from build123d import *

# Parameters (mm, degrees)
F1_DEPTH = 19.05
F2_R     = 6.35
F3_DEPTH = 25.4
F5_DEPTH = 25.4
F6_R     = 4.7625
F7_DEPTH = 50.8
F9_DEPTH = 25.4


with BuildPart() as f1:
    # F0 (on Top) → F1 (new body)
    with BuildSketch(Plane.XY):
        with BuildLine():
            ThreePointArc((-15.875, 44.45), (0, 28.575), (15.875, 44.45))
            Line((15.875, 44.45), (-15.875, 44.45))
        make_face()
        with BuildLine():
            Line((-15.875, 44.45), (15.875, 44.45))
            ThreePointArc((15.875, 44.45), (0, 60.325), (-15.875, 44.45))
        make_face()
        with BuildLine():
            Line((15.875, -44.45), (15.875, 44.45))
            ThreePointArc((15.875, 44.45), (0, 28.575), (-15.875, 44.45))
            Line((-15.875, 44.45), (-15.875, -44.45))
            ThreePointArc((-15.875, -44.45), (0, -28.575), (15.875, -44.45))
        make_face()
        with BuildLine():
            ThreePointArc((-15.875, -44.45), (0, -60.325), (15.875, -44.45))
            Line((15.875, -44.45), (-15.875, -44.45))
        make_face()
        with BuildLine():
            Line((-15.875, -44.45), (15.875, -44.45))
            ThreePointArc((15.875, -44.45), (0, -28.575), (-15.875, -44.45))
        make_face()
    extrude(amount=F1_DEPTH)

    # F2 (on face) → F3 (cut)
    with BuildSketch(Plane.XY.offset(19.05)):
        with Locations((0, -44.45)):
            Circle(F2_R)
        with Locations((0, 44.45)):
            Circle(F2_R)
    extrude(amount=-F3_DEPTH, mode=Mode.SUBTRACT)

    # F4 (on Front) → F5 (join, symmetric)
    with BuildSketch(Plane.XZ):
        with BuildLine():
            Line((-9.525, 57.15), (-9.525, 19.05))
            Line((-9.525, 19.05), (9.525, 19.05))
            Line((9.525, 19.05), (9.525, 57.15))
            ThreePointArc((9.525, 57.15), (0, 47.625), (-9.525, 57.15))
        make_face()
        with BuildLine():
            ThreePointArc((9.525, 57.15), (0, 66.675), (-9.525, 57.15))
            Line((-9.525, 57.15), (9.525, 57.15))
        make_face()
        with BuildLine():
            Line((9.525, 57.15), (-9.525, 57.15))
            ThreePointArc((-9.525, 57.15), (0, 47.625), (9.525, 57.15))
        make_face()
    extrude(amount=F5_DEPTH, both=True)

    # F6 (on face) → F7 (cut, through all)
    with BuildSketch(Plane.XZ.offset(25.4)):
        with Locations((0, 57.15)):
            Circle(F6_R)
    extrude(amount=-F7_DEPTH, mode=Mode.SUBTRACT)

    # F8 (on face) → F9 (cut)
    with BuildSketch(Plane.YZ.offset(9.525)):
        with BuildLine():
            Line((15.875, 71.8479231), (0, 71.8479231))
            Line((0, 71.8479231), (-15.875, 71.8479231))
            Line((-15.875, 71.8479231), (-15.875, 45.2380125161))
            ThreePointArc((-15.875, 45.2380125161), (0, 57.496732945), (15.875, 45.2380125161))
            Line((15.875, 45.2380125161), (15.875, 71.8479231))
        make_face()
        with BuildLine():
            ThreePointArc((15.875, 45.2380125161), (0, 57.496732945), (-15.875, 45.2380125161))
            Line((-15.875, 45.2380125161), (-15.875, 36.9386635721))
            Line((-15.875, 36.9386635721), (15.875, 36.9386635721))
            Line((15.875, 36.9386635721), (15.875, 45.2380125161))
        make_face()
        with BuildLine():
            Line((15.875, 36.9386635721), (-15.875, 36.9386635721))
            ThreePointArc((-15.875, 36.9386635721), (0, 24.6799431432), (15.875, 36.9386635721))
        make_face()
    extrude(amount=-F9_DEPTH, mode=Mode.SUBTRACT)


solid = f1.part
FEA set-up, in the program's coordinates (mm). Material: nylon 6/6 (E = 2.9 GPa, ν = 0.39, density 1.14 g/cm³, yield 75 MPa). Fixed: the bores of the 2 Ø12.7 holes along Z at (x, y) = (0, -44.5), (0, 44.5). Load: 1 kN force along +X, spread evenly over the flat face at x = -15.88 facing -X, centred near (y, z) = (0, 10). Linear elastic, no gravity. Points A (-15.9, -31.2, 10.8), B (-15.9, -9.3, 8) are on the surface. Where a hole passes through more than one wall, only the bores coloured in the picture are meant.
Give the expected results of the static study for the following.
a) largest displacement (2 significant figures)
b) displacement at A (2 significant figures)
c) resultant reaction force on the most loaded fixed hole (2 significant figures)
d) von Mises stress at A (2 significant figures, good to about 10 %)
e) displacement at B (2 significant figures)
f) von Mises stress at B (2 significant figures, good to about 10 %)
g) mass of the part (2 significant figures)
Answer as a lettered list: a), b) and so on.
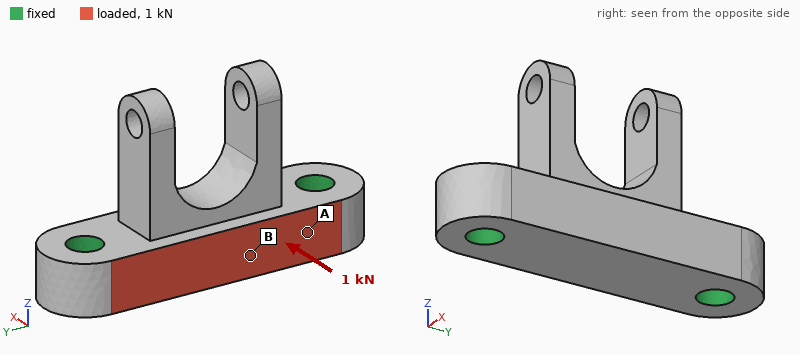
a) 36 µm
b) 17 µm
c) 500 N
d) 0.62 MPa
e) 32 µm
f) 1.4 MPa
g) 96 g
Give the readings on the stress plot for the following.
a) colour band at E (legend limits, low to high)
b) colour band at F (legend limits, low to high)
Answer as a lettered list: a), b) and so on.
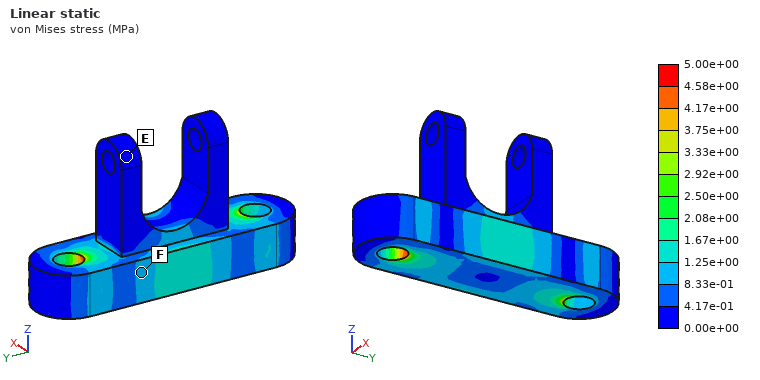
a) 0.00e+00 to 4.17e-01 MPa
b) 8.33e-01 to 1.25e+00 MPa
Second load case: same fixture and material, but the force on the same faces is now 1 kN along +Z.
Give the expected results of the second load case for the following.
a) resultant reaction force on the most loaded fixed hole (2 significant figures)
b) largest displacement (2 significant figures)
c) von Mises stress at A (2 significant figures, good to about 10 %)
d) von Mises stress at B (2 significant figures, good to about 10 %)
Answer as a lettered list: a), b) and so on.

a) 500 N
b) 0.14 mm
c) 4.1 MPa
d) 1.5 MPa
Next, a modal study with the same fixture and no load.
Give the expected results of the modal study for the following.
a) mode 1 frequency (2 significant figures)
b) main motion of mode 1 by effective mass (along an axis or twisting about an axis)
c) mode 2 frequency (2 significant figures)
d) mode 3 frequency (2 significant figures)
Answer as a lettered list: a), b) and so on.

a) 1600 Hz
b) along X
c) 1800 Hz
d) 1800 Hz
